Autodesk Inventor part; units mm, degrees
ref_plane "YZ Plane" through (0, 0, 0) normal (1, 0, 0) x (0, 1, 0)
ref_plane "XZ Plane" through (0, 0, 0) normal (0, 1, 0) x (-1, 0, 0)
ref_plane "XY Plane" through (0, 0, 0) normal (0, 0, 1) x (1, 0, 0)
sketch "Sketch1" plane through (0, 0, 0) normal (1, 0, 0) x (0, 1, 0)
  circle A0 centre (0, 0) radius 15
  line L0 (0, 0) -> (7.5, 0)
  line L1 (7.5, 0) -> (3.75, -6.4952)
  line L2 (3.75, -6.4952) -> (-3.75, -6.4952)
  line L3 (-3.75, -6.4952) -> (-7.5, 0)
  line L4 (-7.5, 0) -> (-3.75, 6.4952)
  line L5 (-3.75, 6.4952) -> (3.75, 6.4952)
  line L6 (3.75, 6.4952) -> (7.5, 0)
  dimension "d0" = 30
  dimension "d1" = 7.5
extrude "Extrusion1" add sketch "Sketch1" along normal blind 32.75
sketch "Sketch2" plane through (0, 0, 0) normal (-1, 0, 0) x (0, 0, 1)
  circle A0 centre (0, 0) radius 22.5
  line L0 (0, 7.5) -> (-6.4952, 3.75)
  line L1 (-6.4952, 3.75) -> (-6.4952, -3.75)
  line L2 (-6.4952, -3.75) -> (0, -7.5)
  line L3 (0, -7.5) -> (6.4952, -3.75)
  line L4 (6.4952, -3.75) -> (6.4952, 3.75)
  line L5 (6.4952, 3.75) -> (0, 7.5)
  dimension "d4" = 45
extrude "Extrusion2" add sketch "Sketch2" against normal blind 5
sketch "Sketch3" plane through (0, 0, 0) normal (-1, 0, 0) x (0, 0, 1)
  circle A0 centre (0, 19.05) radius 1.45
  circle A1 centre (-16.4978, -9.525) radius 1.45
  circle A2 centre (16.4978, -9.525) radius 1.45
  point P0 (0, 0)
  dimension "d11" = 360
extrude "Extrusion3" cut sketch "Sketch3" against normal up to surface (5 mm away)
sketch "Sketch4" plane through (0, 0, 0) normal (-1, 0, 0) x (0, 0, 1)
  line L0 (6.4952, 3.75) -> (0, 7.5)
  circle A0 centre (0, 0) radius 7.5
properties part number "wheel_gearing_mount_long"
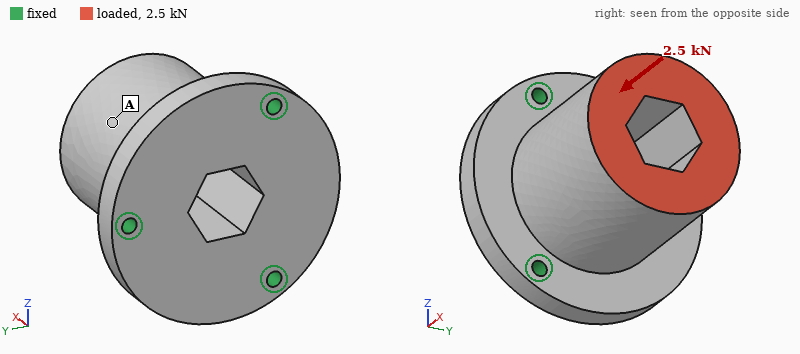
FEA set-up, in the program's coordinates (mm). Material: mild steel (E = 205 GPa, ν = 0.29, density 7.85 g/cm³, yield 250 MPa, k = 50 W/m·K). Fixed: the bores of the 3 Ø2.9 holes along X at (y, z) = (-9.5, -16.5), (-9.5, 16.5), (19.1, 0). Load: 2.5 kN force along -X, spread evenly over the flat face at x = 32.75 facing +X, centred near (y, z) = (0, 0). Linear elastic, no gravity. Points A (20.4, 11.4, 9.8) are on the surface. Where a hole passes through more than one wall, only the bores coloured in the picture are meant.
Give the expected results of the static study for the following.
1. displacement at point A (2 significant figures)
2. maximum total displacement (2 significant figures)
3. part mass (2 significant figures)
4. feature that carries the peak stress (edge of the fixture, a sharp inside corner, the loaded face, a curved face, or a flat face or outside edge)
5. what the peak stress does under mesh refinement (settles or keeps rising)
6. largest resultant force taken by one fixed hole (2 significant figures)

2.5 µm
2.7 µm
180 g
edge of the fixture
keeps rising
880 N
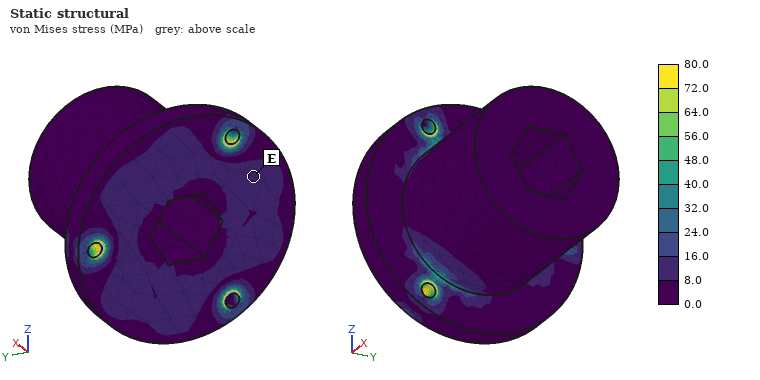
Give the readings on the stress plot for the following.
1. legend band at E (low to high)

8.0 to 16.0 MPa
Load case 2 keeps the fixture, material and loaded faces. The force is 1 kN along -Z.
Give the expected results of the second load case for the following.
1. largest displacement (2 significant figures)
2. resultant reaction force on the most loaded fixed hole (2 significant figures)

8.1 µm
1.1 kN
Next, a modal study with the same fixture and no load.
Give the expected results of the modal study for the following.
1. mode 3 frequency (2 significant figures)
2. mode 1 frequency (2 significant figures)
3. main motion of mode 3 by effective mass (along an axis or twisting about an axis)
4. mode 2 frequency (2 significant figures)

13 kHz
8200 Hz
along X
8200 Hz
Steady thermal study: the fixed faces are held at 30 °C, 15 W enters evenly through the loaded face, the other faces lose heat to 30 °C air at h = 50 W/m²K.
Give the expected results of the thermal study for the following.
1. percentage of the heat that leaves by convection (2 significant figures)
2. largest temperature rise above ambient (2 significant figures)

24 %
21 K
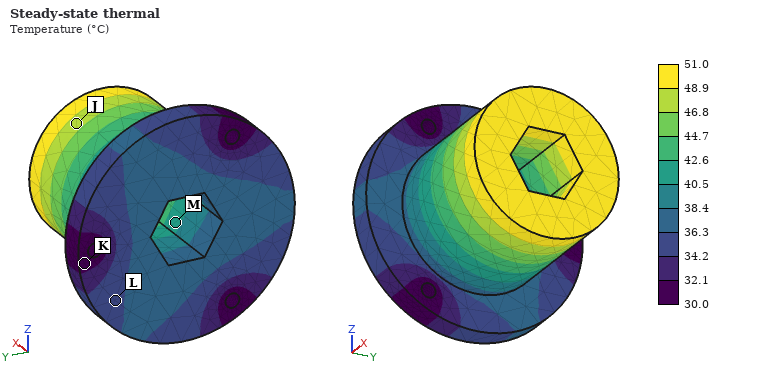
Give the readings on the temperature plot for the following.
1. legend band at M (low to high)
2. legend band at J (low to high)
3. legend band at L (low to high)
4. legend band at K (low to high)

40.5 to 42.6 °C
46.8 to 48.9 °C
34.2 to 36.3 °C
30.0 to 32.1 °C
